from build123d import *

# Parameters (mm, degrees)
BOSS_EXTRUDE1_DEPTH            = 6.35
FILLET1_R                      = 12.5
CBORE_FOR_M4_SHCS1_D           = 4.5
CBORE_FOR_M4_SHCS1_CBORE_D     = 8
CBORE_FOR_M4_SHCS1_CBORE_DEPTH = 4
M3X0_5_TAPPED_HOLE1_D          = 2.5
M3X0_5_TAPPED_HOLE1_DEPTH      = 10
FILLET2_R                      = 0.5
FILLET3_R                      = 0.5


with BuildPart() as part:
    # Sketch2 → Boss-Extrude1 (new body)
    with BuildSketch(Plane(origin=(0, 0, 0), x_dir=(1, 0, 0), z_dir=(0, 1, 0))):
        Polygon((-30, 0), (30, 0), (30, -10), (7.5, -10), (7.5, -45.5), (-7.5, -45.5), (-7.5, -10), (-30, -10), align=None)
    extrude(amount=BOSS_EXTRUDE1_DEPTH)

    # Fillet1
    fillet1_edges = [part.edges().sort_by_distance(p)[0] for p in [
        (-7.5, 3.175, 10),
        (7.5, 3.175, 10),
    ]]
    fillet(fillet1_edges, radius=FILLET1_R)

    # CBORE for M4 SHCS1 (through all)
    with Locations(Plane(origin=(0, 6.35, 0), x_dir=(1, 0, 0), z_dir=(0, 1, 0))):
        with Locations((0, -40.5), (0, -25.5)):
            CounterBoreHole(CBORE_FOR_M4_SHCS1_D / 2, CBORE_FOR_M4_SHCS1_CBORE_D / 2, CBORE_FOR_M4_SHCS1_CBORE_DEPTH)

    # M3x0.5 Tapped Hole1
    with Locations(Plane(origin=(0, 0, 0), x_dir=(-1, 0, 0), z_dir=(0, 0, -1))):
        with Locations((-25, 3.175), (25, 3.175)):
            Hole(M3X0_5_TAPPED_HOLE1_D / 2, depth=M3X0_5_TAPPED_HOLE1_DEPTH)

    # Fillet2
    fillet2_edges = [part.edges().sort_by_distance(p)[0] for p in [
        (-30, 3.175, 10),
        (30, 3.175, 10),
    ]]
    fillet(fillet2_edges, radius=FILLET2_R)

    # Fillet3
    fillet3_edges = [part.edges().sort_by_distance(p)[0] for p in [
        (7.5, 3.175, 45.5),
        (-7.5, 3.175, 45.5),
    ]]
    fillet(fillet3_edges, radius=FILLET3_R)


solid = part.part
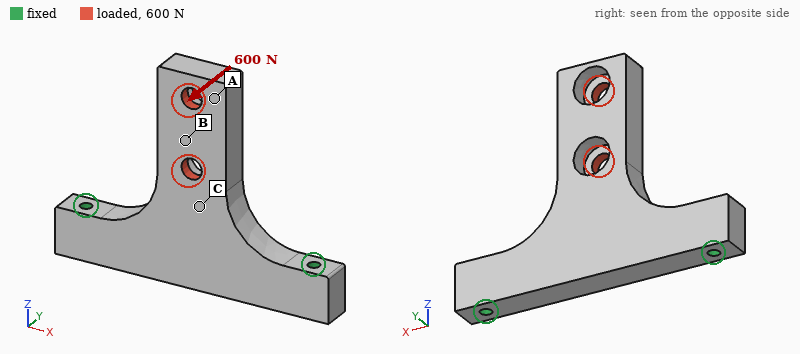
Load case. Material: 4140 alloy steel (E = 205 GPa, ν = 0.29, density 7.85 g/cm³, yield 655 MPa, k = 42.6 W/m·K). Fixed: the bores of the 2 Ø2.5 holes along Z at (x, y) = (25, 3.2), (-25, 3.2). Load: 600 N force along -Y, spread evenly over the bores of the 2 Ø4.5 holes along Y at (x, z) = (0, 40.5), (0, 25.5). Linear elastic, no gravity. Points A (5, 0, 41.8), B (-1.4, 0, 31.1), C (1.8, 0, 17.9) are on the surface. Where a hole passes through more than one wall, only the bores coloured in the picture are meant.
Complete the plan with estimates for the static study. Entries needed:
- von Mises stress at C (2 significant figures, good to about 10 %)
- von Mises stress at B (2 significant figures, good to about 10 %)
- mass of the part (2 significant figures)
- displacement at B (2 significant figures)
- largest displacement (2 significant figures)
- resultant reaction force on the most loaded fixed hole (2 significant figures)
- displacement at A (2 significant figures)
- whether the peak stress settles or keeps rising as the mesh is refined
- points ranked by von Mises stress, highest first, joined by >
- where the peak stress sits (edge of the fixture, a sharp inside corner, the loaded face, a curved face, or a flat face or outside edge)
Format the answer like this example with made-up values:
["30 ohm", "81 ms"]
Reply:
["87 MPa", "35 MPa", "55 g", "0.12 mm", "0.21 mm", "300 N", "0.18 mm", "keeps rising", "C > B > A", "edge of the fixture"]
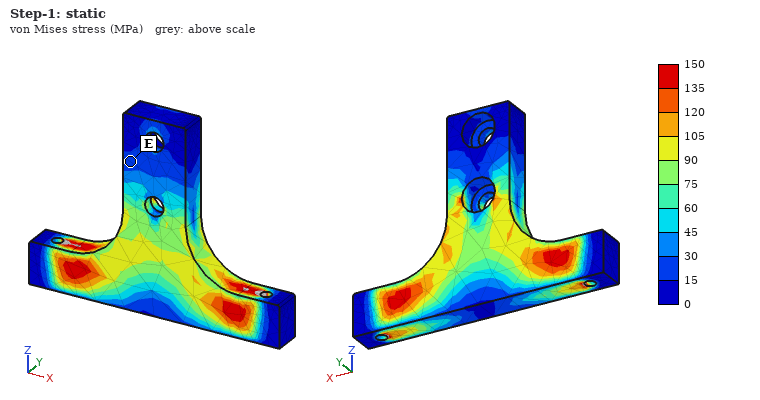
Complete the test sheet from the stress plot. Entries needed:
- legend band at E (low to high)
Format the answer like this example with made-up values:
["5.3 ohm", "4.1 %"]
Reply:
["15 to 30 MPa"]
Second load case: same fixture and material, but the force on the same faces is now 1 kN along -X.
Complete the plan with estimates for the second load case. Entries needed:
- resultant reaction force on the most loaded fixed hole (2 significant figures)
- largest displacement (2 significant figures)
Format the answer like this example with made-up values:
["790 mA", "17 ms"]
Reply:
["860 N", "30 µm"]
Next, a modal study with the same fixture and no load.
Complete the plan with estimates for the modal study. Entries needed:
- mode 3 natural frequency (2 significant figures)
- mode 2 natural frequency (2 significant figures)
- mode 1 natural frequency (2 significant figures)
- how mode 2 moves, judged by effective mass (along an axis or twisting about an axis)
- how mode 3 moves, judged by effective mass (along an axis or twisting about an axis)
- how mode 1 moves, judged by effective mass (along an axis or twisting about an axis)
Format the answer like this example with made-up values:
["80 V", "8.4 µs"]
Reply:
["9600 Hz", "9100 Hz", "2600 Hz", "along X", "along Y", "along Y"]
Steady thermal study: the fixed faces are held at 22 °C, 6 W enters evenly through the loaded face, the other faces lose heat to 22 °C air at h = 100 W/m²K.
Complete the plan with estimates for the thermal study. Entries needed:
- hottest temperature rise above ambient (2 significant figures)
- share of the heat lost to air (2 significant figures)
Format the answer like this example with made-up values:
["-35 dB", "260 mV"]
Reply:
["30 K", "65 %"]
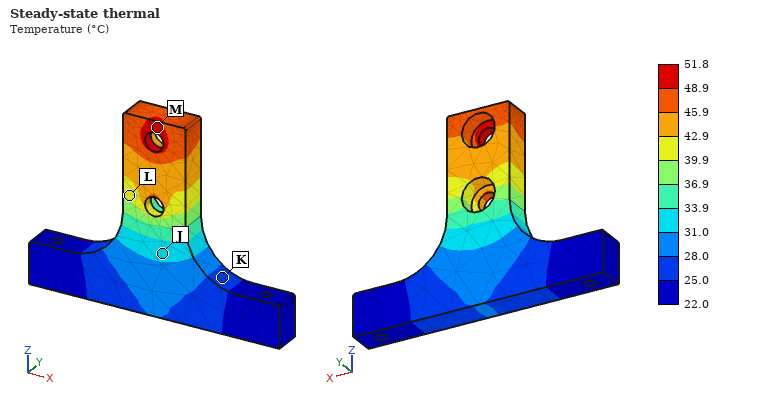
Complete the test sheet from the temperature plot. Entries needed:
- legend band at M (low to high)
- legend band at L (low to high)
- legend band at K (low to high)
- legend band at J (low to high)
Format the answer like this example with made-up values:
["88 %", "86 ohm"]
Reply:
["48.9 to 51.8 °C", "39.9 to 42.9 °C", "25.0 to 28.0 °C", "31.0 to 33.9 °C"]
